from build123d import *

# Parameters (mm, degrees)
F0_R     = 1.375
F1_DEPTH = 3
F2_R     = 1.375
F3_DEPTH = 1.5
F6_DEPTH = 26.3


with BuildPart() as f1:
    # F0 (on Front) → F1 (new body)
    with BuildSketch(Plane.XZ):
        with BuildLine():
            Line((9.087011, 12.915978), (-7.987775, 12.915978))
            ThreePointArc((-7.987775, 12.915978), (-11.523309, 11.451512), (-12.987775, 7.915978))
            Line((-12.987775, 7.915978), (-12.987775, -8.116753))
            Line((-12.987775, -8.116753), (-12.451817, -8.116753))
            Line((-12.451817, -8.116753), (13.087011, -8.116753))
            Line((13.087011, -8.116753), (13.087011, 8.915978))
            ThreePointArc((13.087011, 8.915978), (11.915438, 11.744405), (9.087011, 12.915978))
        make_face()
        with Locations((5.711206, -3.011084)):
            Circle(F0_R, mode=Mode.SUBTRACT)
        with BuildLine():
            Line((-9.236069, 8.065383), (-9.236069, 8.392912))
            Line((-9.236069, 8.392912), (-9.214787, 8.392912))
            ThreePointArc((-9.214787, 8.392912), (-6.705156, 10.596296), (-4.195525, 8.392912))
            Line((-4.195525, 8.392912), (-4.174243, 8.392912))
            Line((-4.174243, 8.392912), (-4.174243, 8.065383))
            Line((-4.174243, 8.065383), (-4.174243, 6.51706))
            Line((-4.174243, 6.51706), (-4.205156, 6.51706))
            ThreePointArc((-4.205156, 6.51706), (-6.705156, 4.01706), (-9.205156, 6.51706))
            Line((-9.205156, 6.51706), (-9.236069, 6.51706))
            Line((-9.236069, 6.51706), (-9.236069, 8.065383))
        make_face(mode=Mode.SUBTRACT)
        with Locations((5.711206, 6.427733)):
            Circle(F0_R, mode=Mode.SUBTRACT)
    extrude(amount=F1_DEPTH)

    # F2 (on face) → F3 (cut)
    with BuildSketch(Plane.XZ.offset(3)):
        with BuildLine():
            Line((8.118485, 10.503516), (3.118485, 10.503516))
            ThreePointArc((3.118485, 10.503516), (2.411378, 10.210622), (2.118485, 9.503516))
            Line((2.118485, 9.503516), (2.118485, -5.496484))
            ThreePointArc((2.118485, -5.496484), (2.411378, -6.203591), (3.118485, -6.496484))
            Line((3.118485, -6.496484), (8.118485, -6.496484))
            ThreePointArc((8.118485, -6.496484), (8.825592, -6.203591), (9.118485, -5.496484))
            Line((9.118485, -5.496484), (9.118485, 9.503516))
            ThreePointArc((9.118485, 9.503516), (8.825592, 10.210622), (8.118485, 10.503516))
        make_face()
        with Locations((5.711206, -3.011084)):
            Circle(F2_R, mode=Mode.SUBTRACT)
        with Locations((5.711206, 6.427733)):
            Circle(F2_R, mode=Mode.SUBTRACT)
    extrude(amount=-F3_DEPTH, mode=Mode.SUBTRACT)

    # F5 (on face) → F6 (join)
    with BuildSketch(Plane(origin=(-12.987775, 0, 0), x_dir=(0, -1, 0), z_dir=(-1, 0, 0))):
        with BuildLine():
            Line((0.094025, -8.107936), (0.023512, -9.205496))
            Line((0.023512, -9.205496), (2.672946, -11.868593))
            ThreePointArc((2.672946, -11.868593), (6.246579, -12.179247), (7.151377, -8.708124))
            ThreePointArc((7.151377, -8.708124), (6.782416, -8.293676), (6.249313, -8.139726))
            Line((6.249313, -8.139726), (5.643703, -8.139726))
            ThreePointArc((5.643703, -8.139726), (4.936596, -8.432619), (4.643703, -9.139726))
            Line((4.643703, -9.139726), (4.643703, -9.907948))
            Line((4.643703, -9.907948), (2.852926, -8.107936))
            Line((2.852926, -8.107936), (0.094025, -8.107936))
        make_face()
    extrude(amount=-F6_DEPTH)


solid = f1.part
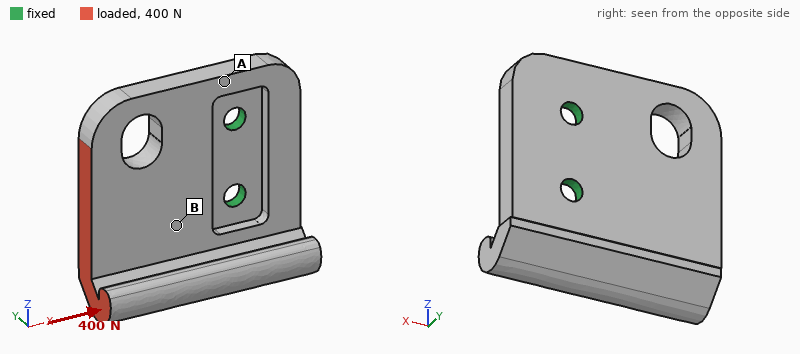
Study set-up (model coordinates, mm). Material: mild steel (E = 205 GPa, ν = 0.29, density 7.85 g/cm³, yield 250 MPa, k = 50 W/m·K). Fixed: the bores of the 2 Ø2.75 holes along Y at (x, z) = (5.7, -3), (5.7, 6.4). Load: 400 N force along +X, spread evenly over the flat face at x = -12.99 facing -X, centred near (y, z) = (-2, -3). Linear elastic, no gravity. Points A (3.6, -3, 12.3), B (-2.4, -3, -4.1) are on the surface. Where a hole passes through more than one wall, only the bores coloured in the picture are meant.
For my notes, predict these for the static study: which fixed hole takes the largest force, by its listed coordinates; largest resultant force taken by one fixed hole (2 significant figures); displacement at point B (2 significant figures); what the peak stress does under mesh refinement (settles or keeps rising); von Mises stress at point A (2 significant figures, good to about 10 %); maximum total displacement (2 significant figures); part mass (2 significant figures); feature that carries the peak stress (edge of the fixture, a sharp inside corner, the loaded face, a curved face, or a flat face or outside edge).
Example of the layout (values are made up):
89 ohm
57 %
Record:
(5.7, -3)
380 N
5.9 µm
keeps rising
15 MPa
16 µm
15 g
edge of the fixture
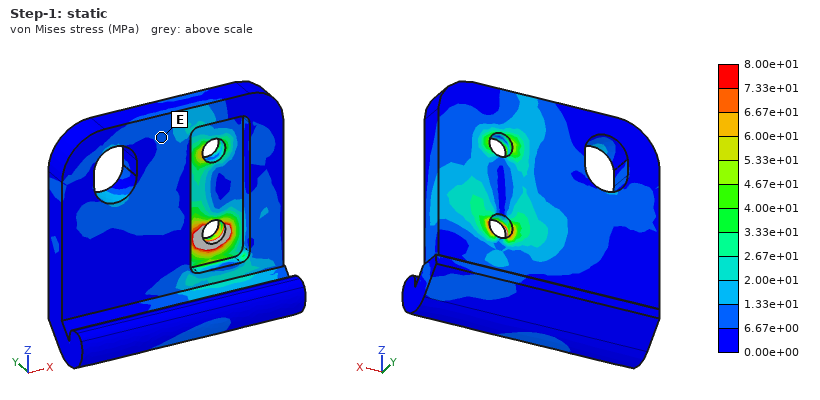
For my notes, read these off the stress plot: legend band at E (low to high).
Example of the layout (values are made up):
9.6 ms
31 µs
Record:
6.67e+00 to 1.33e+01 MPa
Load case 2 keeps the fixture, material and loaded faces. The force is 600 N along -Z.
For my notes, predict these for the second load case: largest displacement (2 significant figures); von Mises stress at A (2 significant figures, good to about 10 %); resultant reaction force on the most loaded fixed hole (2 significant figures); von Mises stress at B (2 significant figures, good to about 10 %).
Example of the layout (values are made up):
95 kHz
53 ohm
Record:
20 µm
17 MPa
1.0 kN
32 MPa
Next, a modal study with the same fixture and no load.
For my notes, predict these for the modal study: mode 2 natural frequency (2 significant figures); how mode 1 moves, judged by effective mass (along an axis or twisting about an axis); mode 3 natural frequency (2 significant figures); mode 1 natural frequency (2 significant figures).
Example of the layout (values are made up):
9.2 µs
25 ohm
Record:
8200 Hz
along Y
13 kHz
4000 Hz
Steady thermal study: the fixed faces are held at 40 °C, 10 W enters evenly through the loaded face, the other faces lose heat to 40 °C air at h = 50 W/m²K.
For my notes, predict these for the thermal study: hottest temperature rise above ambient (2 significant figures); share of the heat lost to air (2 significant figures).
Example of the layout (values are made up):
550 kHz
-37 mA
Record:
58 K
21 %
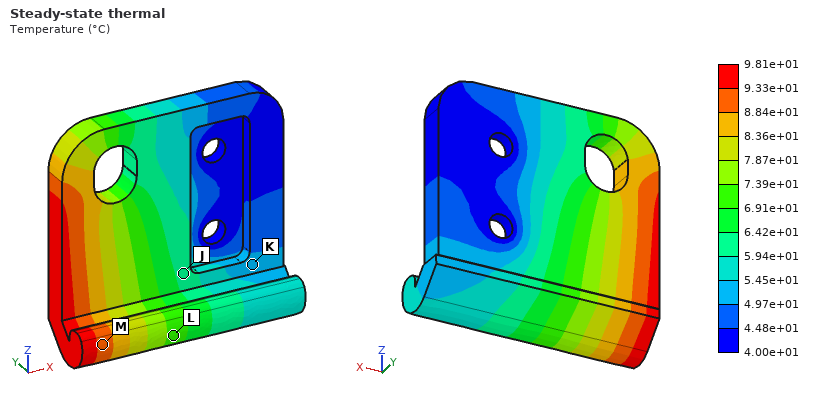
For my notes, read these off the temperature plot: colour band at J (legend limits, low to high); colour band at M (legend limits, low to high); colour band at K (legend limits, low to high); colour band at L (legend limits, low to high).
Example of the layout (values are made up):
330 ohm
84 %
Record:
5.94e+01 to 6.42e+01 °C
8.84e+01 to 9.33e+01 °C
4.97e+01 to 5.45e+01 °C
6.91e+01 to 7.39e+01 °C
